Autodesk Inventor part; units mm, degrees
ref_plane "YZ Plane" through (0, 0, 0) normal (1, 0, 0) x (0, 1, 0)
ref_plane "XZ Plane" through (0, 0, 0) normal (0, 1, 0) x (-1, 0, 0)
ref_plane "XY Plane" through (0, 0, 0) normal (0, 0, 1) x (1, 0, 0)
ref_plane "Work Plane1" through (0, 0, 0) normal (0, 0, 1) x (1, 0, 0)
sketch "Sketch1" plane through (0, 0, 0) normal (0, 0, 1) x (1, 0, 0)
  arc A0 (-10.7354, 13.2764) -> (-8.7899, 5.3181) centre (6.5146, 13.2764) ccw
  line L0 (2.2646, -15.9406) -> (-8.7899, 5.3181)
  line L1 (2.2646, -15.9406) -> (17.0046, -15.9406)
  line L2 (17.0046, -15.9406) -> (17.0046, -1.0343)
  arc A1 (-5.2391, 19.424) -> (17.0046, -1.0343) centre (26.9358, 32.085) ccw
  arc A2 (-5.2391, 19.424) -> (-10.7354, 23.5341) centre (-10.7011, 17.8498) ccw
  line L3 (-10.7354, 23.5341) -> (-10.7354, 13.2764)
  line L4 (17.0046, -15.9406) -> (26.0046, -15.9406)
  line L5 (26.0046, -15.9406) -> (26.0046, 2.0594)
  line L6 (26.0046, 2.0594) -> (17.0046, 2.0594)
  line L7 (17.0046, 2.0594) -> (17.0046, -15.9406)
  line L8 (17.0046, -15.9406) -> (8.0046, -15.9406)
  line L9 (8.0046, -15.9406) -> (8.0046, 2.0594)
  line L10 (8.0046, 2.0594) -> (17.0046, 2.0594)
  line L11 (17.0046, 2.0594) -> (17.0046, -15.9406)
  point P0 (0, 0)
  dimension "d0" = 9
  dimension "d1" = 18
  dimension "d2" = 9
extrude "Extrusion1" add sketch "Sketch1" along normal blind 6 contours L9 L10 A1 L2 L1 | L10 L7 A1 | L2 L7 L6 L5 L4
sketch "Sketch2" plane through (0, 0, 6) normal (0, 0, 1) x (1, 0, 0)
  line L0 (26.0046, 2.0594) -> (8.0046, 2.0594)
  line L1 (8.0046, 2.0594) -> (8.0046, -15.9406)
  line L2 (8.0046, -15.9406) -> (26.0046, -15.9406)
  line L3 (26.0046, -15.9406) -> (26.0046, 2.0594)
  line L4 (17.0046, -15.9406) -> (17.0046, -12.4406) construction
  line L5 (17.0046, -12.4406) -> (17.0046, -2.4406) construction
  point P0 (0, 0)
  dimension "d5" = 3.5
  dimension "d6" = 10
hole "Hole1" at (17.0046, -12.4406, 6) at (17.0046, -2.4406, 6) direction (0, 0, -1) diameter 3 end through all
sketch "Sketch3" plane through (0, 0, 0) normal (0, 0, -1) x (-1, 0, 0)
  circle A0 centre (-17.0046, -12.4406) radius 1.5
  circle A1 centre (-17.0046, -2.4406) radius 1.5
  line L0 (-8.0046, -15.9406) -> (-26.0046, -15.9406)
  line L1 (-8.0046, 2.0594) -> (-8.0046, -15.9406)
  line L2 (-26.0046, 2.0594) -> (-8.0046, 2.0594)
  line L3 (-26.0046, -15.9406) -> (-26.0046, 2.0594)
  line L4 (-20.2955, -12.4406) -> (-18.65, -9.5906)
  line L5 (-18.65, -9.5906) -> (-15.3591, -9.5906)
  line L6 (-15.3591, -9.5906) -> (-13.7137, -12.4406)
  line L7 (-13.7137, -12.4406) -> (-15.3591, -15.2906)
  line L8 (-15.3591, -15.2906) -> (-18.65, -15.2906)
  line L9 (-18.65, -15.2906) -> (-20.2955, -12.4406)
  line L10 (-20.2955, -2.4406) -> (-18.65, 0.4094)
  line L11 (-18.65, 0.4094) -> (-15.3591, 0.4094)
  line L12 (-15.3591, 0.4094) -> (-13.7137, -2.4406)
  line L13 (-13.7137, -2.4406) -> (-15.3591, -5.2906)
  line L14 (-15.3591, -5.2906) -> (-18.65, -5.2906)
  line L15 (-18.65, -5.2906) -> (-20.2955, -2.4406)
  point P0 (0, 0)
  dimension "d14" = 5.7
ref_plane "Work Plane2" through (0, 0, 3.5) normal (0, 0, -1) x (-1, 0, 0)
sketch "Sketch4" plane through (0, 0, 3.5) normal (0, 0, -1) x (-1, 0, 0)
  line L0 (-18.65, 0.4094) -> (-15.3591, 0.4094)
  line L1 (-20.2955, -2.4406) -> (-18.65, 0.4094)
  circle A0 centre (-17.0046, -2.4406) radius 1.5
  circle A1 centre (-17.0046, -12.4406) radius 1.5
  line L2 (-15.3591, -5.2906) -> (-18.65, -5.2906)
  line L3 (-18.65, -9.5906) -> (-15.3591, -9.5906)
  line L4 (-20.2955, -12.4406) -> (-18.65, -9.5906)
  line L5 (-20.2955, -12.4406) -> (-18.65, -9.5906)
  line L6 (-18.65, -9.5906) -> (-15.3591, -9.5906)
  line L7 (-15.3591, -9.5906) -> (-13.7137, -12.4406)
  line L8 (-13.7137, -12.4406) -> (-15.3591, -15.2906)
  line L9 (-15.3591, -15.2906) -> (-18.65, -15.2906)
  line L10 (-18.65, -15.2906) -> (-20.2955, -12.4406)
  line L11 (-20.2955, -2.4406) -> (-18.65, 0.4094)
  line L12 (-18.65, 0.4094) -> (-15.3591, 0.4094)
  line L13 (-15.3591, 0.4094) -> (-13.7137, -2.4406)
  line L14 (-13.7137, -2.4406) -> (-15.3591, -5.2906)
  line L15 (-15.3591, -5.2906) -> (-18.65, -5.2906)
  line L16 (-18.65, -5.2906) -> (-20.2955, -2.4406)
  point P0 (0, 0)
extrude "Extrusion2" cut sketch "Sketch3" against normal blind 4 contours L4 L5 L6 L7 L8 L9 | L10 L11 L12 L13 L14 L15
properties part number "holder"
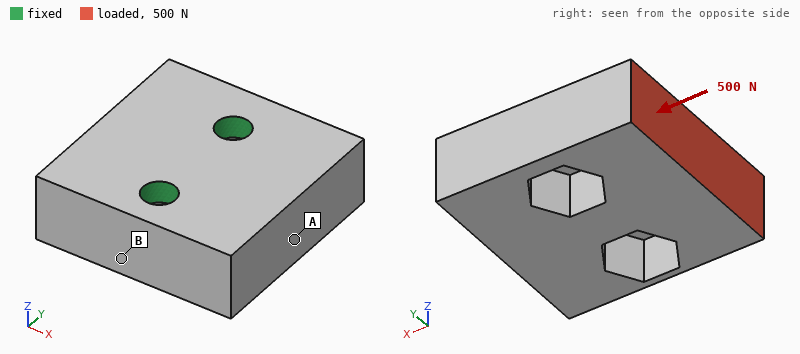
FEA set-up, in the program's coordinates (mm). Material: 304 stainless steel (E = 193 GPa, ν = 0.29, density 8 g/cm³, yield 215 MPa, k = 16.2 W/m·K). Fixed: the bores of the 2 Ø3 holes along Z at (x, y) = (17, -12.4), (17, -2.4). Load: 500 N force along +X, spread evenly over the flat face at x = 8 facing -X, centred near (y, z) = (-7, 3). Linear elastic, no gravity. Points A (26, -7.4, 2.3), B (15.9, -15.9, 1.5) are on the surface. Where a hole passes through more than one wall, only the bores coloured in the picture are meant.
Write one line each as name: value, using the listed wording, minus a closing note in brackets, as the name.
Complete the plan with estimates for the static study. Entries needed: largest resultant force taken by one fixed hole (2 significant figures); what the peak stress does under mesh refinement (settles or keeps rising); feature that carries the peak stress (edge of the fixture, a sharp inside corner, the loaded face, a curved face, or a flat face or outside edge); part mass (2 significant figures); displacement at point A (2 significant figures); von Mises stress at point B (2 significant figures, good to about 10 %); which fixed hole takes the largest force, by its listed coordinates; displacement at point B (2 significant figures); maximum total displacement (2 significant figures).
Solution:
largest resultant force taken by one fixed hole: 270 N
what the peak stress does under mesh refinement: keeps rising
feature that carries the peak stress: edge of the fixture
part mass: 14 g
displacement at point A: 2.3 µm
von Mises stress at point B: 13 MPa
which fixed hole takes the largest force, by its listed coordinates: (17, -2.4)
displacement at point B: 1.1 µm
maximum total displacement: 3.2 µm
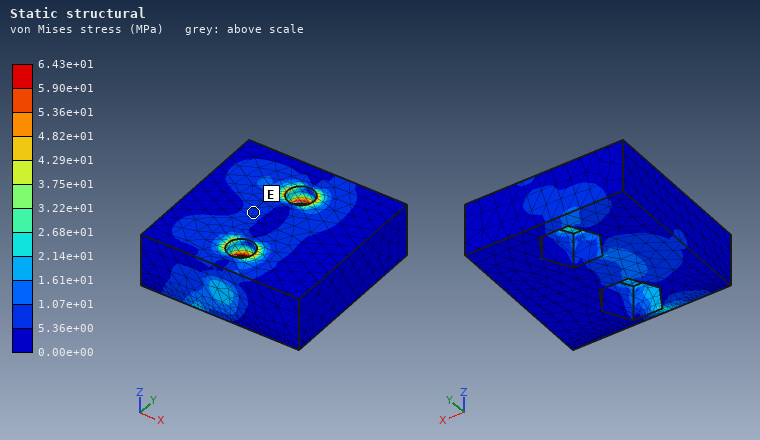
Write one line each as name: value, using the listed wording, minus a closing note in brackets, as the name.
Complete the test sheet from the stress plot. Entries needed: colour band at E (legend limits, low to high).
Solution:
colour band at E: 5.36e+00 to 1.07e+01 MPa
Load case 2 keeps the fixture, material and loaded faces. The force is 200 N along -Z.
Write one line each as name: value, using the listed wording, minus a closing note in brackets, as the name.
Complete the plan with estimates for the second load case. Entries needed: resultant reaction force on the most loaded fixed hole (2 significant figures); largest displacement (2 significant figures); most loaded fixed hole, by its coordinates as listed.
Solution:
resultant reaction force on the most loaded fixed hole: 110 N
largest displacement: 5.4 µm
most loaded fixed hole, by its coordinates as listed: (17, -2.4)
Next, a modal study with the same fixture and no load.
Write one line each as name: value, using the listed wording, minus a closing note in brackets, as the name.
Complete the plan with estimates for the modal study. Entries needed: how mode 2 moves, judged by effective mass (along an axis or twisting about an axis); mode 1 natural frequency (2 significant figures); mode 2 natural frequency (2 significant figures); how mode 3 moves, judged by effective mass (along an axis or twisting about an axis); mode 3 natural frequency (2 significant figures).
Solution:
how mode 2 moves, judged by effective mass: along Z
mode 1 natural frequency: 15 kHz
mode 2 natural frequency: 34 kHz
how mode 3 moves, judged by effective mass: along Y
mode 3 natural frequency: 37 kHz
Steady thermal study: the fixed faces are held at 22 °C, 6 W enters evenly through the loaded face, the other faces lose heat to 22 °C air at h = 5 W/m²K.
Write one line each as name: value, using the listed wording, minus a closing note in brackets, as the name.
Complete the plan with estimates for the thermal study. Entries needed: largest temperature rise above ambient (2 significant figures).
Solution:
largest temperature rise above ambient: 45 K
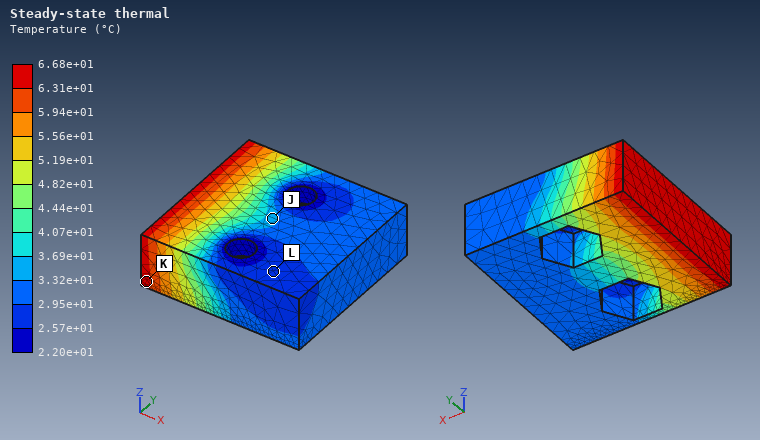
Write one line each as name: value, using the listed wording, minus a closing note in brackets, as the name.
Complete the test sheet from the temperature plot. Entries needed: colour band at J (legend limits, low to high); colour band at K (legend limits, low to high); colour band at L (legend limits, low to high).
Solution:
colour band at J: 3.32e+01 to 3.69e+01 °C
colour band at K: 6.31e+01 to 6.68e+01 °C
colour band at L: 2.57e+01 to 2.95e+01 °C
